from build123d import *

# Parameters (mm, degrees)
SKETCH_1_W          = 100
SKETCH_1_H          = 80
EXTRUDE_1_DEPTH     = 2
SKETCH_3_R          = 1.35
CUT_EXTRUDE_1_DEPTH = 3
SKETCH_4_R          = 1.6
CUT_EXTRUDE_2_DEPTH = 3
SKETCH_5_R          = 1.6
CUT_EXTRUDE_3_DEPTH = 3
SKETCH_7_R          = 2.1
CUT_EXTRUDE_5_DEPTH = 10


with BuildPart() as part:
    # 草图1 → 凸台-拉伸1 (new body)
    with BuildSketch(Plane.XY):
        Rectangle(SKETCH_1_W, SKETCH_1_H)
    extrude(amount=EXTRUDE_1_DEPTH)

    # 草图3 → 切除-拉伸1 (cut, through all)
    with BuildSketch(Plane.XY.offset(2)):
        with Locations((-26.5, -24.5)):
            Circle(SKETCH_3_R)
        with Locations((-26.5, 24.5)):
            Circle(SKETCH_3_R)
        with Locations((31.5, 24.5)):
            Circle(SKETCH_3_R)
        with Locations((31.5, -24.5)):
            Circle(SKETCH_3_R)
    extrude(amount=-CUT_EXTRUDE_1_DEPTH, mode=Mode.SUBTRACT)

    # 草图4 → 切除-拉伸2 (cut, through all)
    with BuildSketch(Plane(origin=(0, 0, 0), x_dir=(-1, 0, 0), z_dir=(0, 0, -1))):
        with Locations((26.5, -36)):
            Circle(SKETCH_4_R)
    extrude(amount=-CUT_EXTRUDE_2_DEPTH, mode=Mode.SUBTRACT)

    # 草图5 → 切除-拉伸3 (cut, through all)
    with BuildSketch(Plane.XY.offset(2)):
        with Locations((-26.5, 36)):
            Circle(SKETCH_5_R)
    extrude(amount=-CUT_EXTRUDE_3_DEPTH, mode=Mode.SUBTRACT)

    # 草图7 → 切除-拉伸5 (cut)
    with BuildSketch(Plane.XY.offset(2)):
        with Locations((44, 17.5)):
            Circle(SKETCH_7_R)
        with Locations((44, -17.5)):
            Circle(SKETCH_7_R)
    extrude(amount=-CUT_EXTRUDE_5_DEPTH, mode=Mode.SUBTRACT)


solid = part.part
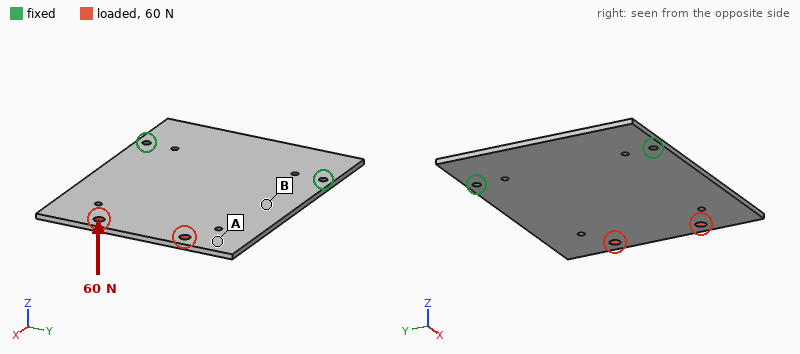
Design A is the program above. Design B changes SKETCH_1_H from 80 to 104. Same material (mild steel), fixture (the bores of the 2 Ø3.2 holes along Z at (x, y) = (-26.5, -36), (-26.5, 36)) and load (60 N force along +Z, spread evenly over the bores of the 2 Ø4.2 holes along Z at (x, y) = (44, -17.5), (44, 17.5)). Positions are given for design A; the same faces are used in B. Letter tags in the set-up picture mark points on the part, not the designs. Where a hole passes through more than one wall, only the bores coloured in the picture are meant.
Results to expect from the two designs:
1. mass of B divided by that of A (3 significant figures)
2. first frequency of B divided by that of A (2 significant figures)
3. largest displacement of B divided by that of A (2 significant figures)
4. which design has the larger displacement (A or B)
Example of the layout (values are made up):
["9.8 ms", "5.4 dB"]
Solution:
["1.30", "1.1", "0.72", "A"]
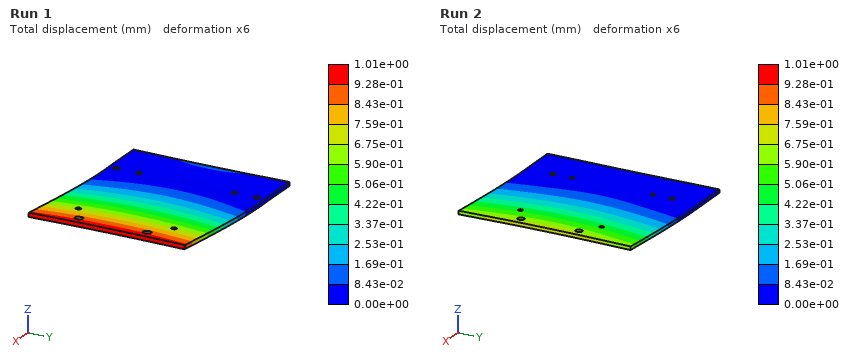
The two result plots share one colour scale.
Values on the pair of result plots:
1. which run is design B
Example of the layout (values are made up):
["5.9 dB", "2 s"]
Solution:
["Run 2"]
